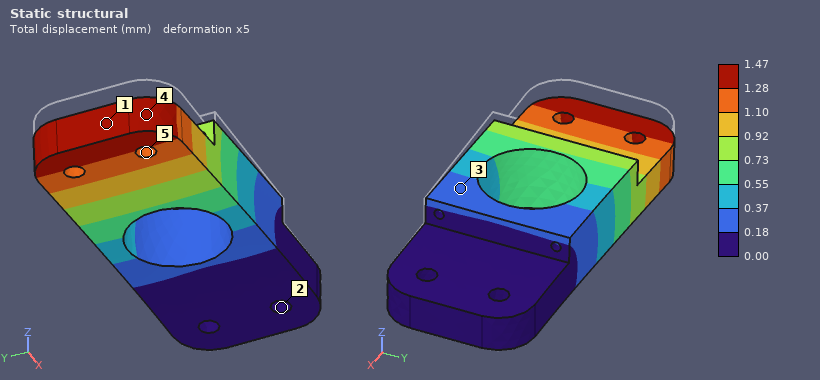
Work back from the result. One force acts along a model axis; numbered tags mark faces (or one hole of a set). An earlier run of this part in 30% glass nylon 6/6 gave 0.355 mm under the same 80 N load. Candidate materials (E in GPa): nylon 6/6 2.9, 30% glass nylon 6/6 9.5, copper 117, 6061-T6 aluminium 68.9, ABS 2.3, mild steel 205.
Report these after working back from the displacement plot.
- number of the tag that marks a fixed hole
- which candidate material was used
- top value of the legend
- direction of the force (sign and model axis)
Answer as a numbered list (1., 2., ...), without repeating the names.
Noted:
1. 2
2. ABS
3. 1.47 mm
4. -Z
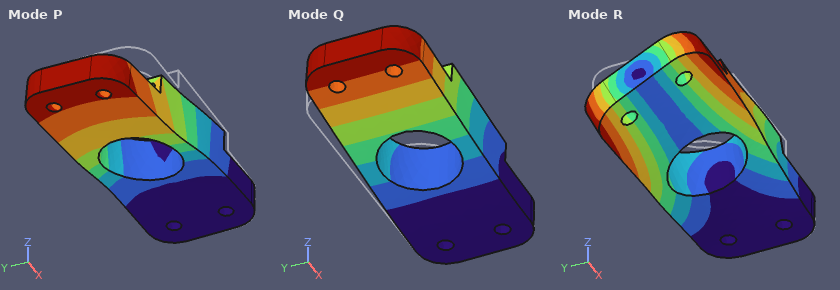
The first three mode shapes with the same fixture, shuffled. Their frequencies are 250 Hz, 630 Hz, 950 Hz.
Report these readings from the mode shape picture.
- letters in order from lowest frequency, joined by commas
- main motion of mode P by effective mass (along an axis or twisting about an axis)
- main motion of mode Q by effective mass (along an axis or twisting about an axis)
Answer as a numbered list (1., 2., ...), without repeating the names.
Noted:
1. Q, P, R
2. along Y
3. along Z
